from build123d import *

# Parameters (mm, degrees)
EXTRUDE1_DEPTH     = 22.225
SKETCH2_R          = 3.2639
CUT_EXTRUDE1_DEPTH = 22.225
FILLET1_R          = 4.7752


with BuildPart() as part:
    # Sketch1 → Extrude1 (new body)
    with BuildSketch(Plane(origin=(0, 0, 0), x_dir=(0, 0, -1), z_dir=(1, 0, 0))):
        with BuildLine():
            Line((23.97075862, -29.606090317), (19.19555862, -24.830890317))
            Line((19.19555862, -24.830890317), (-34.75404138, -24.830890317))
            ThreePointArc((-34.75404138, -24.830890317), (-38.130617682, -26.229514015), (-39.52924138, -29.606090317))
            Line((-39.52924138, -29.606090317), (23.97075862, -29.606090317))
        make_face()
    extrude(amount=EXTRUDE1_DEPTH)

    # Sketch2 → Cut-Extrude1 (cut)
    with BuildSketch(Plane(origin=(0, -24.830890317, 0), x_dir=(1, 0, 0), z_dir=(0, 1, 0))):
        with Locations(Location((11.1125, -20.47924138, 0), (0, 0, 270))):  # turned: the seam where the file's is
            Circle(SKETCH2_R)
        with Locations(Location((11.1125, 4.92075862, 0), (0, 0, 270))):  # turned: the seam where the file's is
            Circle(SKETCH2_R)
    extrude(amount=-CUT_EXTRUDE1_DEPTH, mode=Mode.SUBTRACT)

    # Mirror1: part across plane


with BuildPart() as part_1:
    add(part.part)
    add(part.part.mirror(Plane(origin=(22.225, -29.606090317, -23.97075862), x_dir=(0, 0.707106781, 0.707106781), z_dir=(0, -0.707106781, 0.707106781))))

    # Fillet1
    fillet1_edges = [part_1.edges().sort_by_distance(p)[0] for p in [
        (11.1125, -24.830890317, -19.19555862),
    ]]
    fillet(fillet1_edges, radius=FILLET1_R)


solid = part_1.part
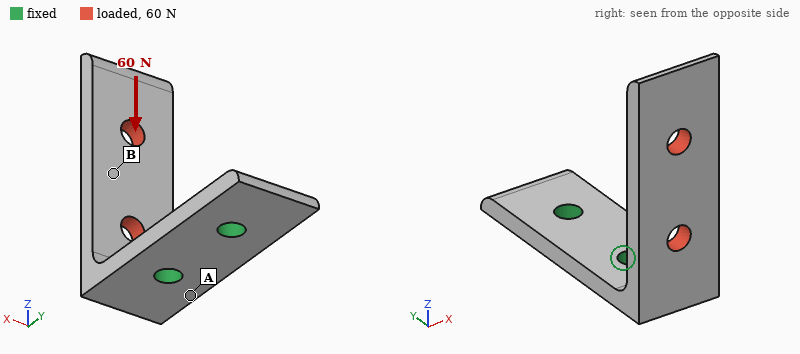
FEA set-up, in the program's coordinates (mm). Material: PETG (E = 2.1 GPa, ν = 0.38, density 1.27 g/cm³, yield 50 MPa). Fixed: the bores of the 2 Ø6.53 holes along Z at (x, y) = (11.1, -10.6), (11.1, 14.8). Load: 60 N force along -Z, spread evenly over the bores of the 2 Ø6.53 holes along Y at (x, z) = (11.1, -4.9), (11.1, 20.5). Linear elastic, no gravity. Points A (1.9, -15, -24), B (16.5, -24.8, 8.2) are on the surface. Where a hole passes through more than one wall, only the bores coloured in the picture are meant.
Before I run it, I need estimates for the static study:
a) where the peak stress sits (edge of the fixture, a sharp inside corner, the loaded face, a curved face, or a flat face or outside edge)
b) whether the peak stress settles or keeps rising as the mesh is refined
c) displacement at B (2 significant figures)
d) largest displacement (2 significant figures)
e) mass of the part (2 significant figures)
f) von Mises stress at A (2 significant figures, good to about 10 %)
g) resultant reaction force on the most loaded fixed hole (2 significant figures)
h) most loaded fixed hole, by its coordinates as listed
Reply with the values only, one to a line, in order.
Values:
edge of the fixture
keeps rising
0.47 mm
0.95 mm
16 g
5.6 MPa
64 N
(11.1, -10.6)
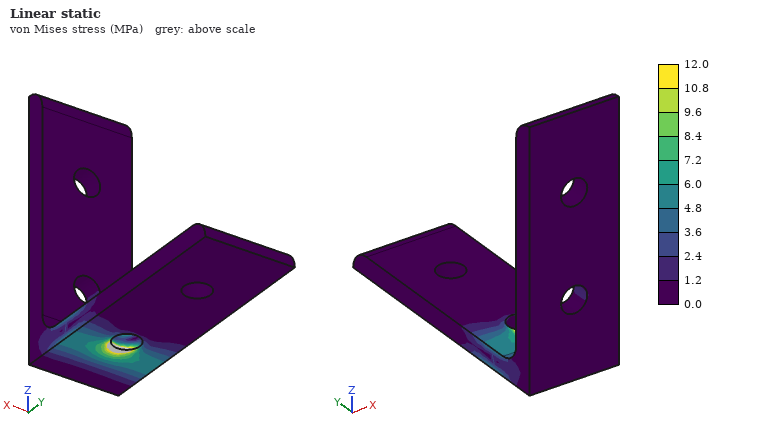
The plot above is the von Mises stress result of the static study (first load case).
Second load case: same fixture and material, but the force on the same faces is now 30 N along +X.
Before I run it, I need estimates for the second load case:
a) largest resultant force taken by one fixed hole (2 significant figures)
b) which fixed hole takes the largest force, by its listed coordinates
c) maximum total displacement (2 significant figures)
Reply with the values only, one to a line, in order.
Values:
40 N
(11.1, -10.6)
1.00 mm
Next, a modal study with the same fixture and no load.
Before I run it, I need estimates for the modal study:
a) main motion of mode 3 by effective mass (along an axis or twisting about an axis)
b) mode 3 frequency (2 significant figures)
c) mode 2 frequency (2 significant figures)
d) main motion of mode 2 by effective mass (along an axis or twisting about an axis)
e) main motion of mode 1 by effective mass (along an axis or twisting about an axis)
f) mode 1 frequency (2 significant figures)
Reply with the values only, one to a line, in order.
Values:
along Z
1100 Hz
380 Hz
along X
along Y
220 Hz
